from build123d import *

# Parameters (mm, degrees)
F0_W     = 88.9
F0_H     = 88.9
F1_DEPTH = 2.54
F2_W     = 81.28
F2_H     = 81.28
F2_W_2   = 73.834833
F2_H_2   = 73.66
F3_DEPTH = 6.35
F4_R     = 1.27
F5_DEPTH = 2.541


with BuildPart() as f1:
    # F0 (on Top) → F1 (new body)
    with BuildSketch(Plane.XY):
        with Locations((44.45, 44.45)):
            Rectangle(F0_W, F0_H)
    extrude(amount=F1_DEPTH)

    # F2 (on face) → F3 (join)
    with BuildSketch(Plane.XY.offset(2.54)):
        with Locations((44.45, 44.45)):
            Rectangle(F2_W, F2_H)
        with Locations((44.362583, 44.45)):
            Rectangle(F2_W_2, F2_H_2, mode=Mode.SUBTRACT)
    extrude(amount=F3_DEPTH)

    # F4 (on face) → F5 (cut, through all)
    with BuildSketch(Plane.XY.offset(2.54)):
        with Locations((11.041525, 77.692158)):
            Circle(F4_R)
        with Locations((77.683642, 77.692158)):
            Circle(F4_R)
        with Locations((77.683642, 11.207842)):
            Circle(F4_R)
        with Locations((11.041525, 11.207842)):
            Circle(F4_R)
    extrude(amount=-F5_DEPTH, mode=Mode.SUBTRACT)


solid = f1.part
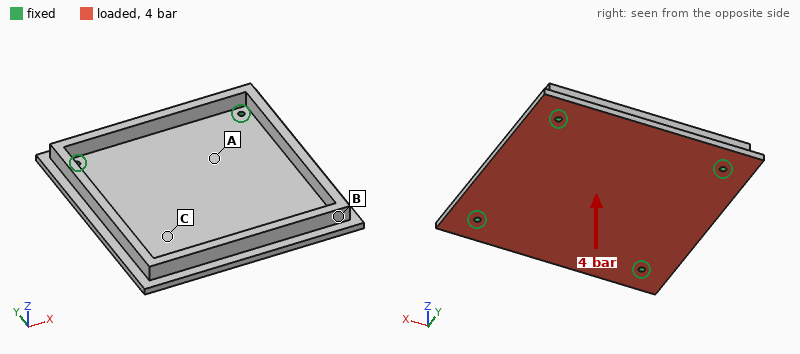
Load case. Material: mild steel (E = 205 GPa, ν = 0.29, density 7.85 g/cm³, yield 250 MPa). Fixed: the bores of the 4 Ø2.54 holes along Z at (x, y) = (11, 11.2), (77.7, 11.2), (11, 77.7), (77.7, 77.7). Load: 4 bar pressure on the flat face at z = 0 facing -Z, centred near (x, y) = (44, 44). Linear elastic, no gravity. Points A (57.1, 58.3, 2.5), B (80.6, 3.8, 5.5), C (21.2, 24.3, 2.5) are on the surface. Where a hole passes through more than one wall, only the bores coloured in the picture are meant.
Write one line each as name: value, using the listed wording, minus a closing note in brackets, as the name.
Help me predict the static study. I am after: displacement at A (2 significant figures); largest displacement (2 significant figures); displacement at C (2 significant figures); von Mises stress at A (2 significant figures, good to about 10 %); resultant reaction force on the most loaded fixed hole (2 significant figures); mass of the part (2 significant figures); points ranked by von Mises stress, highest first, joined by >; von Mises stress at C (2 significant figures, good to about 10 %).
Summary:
displacement at A: 0.086 mm
largest displacement: 0.12 mm
displacement at C: 0.046 mm
von Mises stress at A: 47 MPa
resultant reaction force on the most loaded fixed hole: 870 N
mass of the part: 220 g
points ranked by von Mises stress, highest first, joined by >: A > C > B
von Mises stress at C: 25 MPa
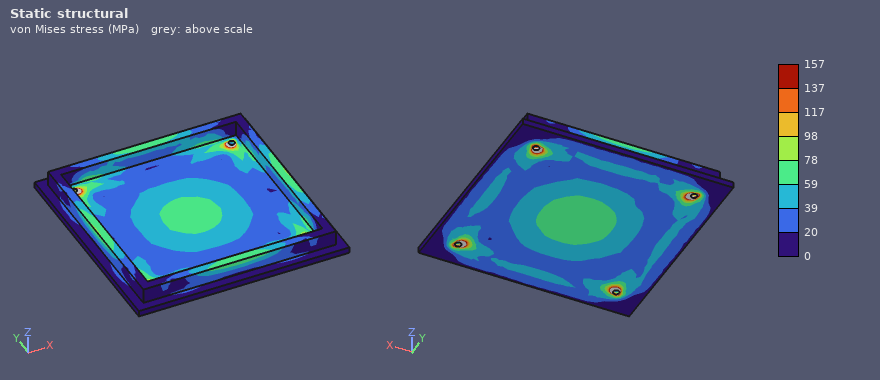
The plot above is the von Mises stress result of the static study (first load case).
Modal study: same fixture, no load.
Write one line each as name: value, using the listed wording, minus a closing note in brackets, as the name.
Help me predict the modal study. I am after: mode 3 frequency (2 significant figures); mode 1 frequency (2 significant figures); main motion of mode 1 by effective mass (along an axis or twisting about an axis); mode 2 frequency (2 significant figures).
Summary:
mode 3 frequency: 4800 Hz
mode 1 frequency: 2600 Hz
main motion of mode 1 by effective mass: along Z
mode 2 frequency: 4700 Hz
